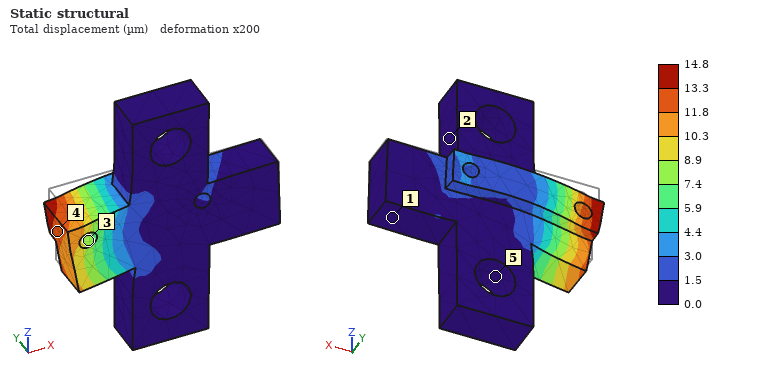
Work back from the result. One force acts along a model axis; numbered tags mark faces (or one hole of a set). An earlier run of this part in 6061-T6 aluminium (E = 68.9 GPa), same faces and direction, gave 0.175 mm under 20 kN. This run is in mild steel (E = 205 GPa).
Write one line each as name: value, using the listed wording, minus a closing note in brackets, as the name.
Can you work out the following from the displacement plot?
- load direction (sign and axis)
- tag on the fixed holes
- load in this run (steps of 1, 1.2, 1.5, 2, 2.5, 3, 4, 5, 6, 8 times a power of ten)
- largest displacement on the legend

load direction: -Z
tag on the fixed holes: 5
load in this run: 5 kN
largest displacement on the legend: 14.8 µm
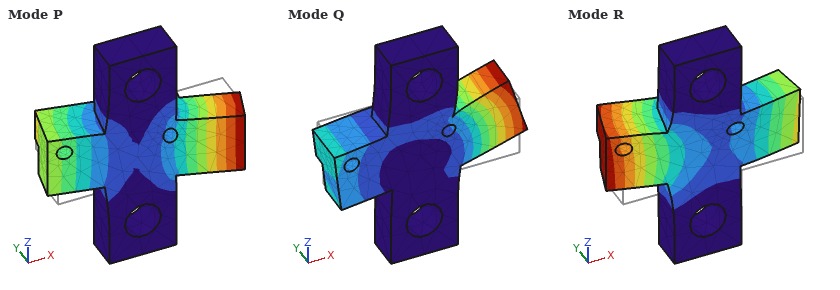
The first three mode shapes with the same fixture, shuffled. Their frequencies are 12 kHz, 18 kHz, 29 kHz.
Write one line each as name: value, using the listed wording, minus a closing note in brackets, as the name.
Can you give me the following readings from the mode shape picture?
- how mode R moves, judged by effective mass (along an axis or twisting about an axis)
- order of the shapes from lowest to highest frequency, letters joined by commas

how mode R moves, judged by effective mass: along Y
order of the shapes from lowest to highest frequency, letters joined by commas: P, R, Q
